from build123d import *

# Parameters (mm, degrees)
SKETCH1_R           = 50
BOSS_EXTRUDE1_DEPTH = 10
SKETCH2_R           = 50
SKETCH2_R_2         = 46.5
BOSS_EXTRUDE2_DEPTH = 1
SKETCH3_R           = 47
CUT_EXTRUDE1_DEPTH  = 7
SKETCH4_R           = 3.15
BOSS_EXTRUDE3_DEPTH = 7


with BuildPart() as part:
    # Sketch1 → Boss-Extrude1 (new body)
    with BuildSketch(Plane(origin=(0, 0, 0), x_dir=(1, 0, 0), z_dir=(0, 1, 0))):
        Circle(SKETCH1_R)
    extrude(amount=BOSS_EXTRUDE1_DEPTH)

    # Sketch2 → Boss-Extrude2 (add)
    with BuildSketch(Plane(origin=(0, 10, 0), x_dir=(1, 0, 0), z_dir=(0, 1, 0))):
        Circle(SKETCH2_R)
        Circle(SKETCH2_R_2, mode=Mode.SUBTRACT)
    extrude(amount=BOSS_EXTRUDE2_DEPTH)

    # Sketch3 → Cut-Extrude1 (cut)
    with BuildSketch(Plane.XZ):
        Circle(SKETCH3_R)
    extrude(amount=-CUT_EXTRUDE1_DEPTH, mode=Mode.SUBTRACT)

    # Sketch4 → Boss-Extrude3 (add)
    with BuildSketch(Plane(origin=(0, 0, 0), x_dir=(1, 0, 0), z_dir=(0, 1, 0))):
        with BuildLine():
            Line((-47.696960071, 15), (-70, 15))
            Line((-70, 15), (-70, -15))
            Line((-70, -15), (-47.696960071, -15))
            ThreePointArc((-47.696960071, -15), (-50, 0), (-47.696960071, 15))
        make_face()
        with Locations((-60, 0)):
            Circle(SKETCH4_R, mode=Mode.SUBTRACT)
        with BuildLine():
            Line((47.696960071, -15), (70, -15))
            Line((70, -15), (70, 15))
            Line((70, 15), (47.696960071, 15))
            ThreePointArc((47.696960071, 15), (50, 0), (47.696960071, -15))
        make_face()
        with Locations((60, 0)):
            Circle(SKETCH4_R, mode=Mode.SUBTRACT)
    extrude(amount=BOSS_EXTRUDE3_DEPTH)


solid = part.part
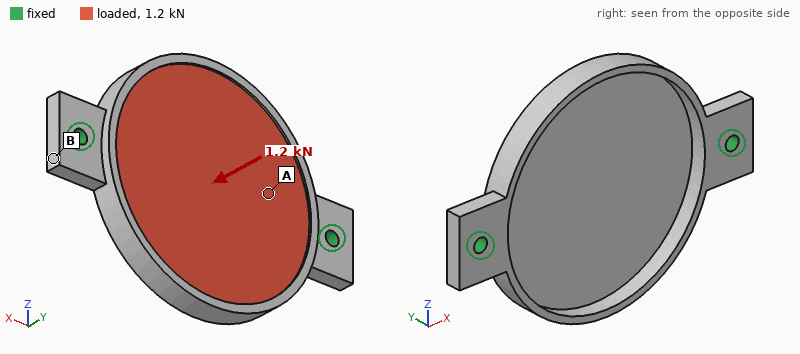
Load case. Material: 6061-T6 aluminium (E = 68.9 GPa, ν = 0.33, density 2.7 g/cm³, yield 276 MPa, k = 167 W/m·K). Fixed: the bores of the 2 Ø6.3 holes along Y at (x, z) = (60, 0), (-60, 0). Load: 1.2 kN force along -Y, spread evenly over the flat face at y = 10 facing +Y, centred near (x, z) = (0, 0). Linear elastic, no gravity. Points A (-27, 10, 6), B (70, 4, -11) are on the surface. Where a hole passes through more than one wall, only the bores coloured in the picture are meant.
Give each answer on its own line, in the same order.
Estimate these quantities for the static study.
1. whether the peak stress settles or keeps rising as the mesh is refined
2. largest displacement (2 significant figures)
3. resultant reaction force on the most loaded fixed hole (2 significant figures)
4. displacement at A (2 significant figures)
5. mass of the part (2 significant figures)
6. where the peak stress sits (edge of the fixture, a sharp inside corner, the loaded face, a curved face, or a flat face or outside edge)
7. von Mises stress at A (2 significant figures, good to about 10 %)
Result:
keeps rising
0.18 mm
1.4 kN
0.10 mm
110 g
edge of the fixture
14 MPa
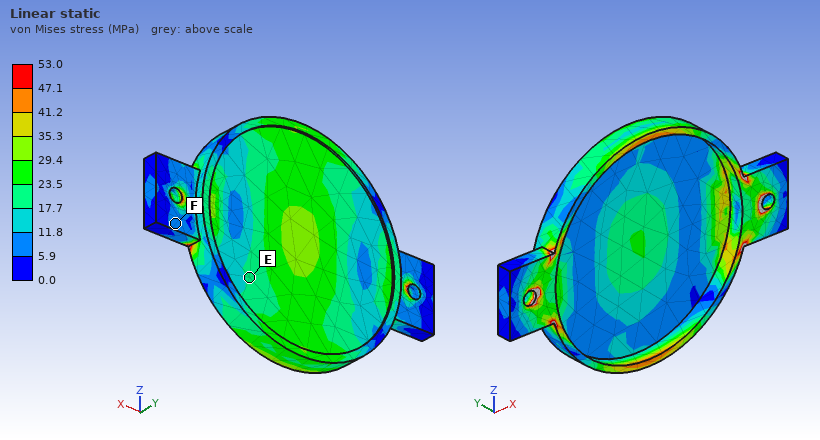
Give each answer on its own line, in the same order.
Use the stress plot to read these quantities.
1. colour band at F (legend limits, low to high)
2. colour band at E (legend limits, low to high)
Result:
5.9 to 11.8 MPa
17.7 to 23.5 MPa
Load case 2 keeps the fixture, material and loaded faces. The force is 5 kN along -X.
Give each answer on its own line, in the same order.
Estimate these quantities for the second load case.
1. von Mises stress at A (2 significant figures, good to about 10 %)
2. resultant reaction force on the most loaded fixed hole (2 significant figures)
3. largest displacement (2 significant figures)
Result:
12 MPa
2.5 kN
33 µm
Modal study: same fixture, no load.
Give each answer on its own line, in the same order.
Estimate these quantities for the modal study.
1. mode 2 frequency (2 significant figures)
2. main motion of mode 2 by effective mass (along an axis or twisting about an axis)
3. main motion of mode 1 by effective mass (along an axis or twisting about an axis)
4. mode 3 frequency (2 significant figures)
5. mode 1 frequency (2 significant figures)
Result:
1700 Hz
along Y
twisting about X
3200 Hz
1500 Hz
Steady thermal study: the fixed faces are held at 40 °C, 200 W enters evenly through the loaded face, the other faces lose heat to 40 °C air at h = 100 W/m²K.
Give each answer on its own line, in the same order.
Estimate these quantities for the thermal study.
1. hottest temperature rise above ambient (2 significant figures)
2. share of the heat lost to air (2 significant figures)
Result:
79 K
45 %
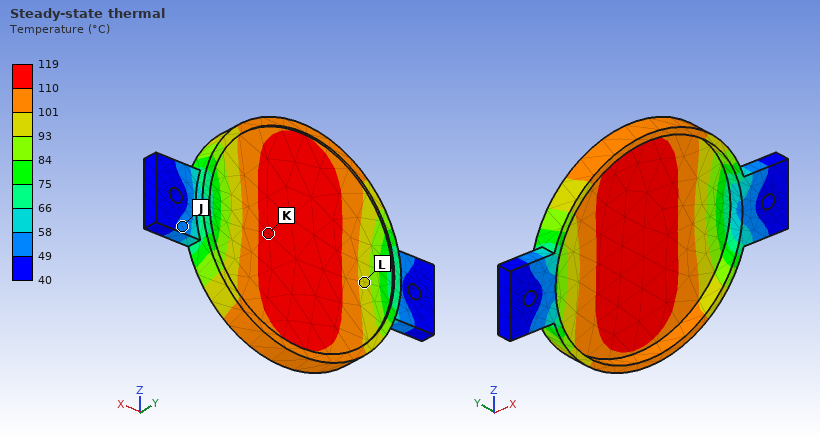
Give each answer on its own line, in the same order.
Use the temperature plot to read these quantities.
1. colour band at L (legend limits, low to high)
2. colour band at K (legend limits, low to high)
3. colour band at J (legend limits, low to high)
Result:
93 to 101 °C
110 to 119 °C
49 to 58 °C
